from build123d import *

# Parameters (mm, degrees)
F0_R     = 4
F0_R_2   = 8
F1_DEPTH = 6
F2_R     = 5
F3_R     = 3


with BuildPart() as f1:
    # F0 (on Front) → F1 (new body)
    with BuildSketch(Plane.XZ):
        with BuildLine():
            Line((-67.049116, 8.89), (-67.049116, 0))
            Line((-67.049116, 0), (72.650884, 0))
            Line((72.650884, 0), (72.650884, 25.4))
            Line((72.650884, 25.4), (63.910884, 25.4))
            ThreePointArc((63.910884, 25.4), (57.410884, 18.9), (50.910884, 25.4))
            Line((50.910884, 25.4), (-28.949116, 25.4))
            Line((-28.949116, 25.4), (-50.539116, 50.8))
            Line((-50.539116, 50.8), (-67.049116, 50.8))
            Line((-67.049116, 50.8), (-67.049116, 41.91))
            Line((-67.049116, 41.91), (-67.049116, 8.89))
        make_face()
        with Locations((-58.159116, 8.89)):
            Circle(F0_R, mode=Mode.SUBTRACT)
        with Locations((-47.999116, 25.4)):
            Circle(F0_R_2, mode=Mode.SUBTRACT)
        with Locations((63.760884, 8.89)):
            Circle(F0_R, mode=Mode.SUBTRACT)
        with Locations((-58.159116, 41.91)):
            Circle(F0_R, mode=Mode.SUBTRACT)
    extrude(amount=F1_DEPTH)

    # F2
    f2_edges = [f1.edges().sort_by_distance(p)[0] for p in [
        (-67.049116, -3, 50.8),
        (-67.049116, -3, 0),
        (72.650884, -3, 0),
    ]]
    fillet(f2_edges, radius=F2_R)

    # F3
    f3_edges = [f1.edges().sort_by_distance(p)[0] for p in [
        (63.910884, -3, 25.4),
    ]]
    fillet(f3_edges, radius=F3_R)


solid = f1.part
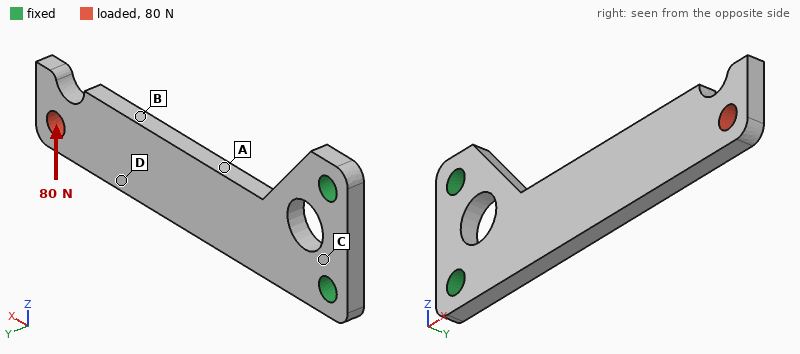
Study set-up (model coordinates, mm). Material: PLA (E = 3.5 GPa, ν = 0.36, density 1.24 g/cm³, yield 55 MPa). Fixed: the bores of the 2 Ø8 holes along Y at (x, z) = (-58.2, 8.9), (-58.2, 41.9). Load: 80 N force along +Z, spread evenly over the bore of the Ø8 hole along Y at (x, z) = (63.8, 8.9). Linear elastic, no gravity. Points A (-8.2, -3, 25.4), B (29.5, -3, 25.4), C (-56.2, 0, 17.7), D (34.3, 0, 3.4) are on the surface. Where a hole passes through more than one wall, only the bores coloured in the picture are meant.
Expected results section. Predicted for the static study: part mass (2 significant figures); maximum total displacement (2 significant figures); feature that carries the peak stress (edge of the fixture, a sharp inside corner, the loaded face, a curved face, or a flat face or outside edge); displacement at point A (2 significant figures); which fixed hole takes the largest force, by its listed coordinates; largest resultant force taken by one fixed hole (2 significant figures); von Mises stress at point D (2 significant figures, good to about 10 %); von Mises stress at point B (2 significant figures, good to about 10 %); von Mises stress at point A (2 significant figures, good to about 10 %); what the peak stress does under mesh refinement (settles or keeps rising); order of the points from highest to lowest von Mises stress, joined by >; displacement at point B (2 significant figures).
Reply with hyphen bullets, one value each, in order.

- 28 g
- 1.5 mm
- a sharp inside corner
- 0.26 mm
- (-58.2, 41.9)
- 300 N
- 2.8 MPa
- 4.2 MPa
- 8.8 MPa
- keeps rising
- A > B > D > C
- 0.76 mm
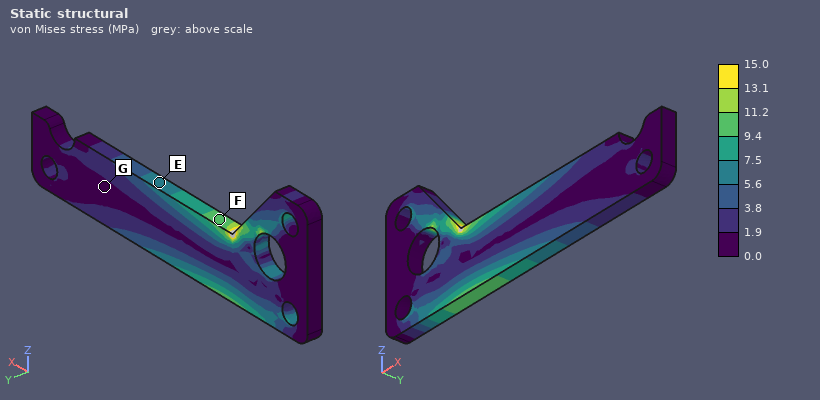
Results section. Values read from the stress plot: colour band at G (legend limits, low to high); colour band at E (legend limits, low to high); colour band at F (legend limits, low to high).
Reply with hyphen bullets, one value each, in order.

- 0.0 to 1.9 MPa
- 5.6 to 7.5 MPa
- 9.4 to 11.2 MPa
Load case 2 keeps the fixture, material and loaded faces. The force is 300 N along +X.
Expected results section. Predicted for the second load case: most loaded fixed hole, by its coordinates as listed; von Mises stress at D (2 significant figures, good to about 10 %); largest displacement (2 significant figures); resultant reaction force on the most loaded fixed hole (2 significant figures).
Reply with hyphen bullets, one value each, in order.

- (-58.2, 8.9)
- 3.3 MPa
- 0.31 mm
- 290 N
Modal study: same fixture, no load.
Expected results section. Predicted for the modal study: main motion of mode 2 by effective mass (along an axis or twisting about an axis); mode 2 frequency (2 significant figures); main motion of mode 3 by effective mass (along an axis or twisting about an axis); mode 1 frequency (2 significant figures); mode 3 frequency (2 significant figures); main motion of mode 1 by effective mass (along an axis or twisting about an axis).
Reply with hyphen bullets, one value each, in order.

- along Z
- 500 Hz
- along Y
- 110 Hz
- 630 Hz
- along Y
